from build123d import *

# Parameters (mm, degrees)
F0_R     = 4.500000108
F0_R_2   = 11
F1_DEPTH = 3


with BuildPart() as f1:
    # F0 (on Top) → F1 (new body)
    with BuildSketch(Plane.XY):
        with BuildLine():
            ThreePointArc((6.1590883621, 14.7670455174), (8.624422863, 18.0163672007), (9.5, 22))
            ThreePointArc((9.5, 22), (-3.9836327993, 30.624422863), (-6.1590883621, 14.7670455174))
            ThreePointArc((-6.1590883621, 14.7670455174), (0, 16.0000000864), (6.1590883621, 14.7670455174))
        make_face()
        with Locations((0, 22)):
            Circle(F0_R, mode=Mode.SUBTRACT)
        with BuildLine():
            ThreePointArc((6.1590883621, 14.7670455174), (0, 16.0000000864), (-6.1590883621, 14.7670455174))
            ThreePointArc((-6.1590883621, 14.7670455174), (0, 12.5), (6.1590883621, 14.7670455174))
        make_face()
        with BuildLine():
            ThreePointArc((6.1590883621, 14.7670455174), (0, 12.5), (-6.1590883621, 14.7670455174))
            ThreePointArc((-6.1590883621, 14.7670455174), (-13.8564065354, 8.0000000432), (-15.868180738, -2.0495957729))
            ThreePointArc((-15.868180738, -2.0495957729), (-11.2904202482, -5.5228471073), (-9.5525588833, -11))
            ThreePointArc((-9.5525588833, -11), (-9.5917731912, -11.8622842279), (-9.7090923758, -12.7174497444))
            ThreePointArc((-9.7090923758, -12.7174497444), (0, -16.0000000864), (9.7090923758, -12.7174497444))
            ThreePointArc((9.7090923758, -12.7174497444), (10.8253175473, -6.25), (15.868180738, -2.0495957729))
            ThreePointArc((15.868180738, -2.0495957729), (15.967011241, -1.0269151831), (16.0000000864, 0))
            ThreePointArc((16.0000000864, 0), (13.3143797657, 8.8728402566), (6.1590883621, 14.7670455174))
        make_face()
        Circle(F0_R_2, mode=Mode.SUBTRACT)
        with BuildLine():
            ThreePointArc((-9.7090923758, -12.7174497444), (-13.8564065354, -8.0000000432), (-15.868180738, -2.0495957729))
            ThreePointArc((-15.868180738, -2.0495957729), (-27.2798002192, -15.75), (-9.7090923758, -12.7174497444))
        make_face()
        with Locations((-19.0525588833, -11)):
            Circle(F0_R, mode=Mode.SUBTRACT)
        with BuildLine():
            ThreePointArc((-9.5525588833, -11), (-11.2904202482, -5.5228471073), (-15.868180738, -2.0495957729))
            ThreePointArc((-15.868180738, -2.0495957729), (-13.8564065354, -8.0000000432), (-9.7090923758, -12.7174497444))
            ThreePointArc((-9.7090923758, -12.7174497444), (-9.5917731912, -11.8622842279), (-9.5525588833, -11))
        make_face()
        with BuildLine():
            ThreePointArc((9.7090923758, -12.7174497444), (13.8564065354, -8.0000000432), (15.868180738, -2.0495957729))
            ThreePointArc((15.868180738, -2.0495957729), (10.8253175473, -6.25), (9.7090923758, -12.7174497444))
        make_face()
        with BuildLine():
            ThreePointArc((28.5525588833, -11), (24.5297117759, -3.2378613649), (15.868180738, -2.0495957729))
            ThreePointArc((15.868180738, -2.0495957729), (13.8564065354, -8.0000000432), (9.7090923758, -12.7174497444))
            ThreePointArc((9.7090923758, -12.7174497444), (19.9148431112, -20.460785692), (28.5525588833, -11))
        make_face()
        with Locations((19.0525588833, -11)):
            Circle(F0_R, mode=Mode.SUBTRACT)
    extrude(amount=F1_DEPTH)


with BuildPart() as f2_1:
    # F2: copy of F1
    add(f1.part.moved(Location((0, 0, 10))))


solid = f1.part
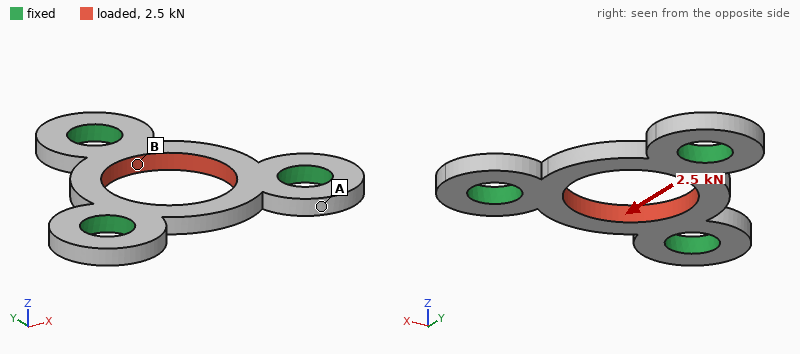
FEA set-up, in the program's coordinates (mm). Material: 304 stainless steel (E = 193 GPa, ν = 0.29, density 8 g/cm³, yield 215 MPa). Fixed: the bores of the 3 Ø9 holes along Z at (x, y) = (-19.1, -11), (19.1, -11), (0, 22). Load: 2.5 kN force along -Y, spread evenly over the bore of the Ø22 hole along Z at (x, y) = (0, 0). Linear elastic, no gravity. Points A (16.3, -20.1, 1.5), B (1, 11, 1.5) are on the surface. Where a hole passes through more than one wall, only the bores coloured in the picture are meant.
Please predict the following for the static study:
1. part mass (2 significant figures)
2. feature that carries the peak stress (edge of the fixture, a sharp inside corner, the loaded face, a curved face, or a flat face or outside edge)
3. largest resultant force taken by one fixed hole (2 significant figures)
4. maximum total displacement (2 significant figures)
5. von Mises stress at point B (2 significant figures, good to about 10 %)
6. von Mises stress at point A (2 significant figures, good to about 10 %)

24 g
edge of the fixture
910 N
6.0 µm
41 MPa
8.7 MPa
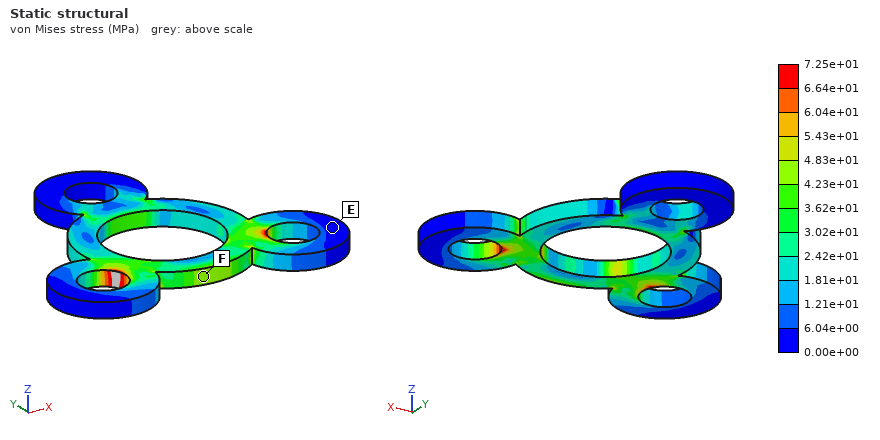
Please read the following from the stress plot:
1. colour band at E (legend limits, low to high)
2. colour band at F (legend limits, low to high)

0.00e+00 to 6.04e+00 MPa
4.23e+01 to 4.83e+01 MPa
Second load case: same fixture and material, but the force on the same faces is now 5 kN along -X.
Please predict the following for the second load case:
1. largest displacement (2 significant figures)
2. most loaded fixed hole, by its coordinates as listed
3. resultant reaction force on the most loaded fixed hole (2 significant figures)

11 µm
(0, 22)
2.0 kN
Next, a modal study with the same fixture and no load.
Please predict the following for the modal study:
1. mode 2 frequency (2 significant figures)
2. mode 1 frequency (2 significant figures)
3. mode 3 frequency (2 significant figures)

18 kHz
18 kHz
18 kHz
